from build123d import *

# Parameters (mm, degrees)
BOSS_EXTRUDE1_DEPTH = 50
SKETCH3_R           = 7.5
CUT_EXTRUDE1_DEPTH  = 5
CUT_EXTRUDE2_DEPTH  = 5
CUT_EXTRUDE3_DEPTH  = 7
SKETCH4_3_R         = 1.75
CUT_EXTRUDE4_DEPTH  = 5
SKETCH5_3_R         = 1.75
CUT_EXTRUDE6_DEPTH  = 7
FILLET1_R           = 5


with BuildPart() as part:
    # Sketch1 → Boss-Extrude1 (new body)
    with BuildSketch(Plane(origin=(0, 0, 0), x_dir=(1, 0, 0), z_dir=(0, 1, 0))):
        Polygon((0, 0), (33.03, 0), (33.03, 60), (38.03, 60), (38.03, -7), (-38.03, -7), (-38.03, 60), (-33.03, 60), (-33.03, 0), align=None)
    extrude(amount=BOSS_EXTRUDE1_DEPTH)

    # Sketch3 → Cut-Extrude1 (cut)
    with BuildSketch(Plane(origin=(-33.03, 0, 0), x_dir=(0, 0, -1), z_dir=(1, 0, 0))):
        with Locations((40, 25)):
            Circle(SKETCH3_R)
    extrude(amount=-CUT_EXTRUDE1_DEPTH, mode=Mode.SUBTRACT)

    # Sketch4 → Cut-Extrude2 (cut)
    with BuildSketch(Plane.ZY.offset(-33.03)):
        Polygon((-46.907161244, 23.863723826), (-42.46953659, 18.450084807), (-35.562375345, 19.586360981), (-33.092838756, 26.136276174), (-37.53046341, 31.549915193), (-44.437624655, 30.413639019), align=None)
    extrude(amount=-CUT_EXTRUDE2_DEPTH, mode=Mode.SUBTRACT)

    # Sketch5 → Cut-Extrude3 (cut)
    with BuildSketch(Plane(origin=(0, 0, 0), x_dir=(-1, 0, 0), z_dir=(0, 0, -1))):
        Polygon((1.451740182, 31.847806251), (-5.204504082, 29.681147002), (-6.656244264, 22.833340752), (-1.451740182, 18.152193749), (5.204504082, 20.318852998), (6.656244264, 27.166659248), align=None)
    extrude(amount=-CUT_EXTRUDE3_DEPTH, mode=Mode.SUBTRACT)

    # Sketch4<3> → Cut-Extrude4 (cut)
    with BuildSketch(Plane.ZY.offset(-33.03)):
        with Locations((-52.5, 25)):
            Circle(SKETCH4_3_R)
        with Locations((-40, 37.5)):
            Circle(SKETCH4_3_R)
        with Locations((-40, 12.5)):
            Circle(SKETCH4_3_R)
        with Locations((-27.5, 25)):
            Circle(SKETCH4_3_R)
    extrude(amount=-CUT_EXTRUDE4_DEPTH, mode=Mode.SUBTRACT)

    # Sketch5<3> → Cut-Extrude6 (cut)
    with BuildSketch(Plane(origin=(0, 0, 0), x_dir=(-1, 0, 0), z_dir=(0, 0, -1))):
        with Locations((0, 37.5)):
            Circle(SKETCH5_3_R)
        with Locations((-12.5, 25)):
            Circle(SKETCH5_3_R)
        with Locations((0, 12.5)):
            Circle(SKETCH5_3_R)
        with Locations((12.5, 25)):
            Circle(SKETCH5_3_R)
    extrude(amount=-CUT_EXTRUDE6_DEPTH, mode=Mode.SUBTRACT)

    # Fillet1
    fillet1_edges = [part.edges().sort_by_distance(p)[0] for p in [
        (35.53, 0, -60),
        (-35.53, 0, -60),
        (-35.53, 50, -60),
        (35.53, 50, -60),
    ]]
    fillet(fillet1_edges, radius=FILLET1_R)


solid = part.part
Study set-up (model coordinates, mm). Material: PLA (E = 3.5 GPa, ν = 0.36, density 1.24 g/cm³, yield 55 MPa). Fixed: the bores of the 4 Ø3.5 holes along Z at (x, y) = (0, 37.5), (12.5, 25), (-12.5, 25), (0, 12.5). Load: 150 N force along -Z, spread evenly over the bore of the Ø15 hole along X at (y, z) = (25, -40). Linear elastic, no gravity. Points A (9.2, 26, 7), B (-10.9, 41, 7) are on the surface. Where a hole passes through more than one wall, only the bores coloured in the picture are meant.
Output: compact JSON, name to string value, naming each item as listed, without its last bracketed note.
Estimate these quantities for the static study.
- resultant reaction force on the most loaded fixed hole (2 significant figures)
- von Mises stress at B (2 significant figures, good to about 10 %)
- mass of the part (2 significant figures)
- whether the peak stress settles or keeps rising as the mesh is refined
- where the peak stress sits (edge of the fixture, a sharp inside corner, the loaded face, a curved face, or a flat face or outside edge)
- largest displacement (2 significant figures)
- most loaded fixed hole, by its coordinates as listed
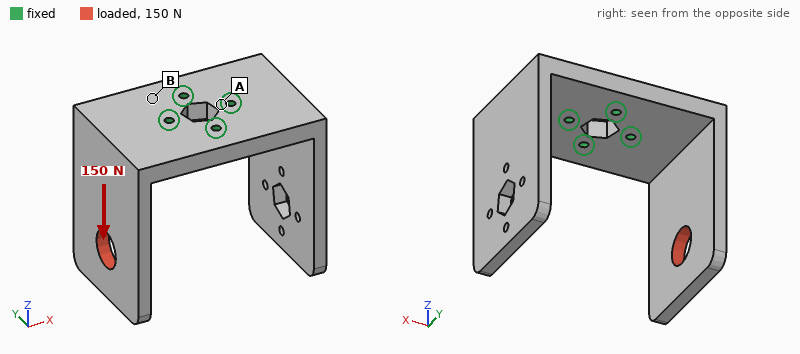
{"resultant reaction force on the most loaded fixed hole": "230 N", "von Mises stress at B": "4.3 MPa", "mass of the part": "67 g", "whether the peak stress settles or keeps rising as the mesh is refined": "keeps rising", "where the peak stress sits": "edge of the fixture", "largest displacement": "0.69 mm", "most loaded fixed hole, by its coordinates as listed": "(-12.5, 25)"}
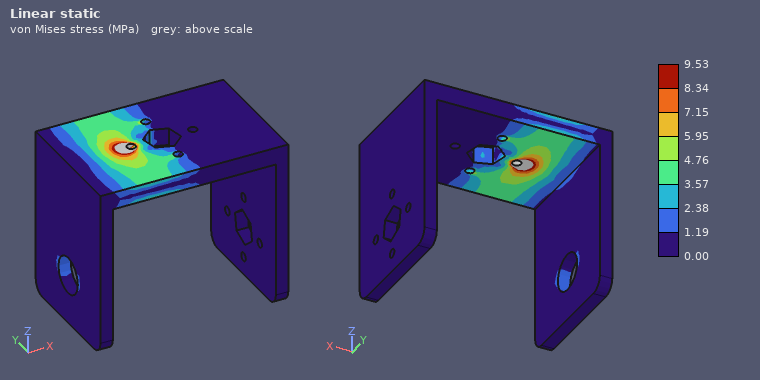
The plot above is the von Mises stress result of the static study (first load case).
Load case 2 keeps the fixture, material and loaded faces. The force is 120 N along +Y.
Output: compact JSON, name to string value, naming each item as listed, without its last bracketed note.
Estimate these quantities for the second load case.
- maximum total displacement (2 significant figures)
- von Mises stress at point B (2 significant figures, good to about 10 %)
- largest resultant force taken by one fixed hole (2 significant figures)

{"maximum total displacement": "1.2 mm", "von Mises stress at point B": "7.5 MPa", "largest resultant force taken by one fixed hole": "130 N"}
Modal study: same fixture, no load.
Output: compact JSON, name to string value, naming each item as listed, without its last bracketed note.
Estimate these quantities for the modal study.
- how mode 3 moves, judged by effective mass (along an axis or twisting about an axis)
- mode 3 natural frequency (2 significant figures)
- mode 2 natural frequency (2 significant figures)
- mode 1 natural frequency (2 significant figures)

{"how mode 3 moves, judged by effective mass": "twisting about Z", "mode 3 natural frequency": "500 Hz", "mode 2 natural frequency": "290 Hz", "mode 1 natural frequency": "290 Hz"}
